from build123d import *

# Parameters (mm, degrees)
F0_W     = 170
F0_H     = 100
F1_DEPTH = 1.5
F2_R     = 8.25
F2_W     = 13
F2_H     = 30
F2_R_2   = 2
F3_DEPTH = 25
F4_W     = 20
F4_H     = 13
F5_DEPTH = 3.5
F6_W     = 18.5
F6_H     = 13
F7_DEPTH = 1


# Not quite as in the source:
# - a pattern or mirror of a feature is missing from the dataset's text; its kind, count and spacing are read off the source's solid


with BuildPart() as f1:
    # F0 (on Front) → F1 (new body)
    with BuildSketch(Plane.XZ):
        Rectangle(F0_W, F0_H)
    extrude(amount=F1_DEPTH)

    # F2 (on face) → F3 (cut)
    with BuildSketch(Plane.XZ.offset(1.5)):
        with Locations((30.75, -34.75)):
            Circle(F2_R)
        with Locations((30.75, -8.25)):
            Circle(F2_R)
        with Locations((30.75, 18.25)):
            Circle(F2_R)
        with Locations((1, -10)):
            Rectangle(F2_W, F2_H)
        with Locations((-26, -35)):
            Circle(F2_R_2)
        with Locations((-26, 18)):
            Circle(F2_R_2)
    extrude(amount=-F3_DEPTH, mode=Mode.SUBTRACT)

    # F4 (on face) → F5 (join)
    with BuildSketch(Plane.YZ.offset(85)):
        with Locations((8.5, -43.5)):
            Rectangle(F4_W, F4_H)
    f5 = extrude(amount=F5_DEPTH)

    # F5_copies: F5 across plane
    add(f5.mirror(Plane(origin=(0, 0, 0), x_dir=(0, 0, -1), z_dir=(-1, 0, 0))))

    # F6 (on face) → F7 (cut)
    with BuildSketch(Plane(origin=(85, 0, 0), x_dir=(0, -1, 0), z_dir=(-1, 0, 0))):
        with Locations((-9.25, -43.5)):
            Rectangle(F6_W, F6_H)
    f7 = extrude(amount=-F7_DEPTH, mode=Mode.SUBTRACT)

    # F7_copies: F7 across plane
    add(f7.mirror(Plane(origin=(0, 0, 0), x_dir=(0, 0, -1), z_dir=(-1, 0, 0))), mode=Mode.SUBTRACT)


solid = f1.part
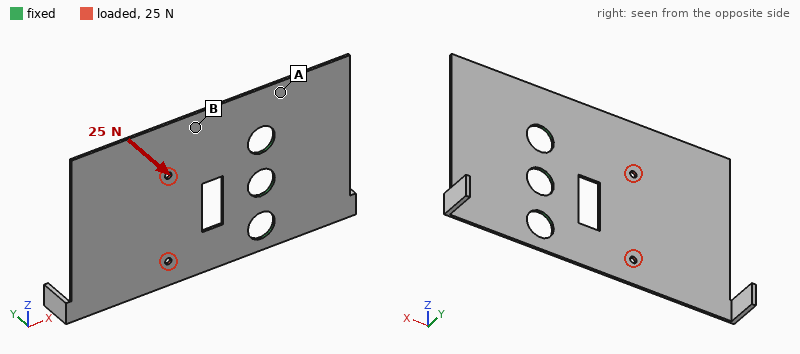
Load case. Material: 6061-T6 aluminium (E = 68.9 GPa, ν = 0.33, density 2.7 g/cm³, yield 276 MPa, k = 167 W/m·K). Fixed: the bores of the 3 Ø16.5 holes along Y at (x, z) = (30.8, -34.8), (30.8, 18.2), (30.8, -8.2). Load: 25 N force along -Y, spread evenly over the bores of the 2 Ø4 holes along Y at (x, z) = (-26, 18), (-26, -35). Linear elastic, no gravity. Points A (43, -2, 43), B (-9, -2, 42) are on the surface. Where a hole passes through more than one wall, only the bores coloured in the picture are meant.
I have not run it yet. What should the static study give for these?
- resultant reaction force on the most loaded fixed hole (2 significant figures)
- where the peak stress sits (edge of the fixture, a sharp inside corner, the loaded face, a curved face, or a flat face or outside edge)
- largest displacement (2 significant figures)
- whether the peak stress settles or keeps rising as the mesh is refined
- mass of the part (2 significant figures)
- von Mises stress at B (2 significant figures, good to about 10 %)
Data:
11 N
a sharp inside corner
2.1 mm
keeps rising
68 g
15 MPa
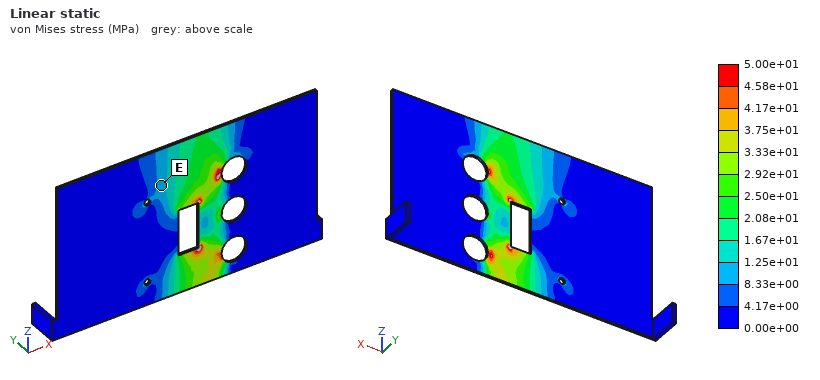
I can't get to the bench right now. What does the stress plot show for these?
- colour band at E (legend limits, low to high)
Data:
8.33e+00 to 1.25e+01 MPa
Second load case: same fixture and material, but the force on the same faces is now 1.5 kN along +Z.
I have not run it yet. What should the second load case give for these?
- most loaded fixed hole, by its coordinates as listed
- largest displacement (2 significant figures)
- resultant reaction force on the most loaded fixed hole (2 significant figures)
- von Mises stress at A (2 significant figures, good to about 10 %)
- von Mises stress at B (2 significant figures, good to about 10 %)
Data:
(30.8, 18.2)
84 µm
1.3 kN
14 MPa
13 MPa
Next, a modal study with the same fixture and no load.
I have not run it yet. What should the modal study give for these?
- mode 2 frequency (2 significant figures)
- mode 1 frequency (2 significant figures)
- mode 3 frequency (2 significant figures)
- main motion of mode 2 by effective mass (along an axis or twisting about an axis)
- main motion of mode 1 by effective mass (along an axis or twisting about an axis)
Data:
230 Hz
86 Hz
430 Hz
twisting about X
along Y
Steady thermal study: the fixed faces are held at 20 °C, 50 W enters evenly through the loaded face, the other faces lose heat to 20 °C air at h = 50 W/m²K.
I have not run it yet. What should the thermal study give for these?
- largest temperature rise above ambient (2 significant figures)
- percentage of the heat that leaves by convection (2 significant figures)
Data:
79 K
68 %
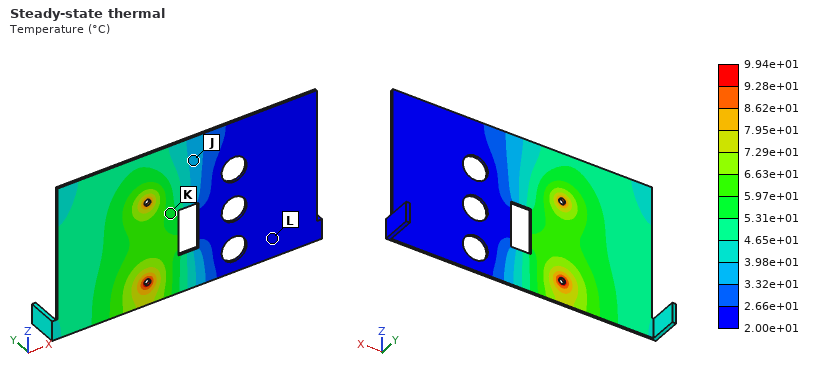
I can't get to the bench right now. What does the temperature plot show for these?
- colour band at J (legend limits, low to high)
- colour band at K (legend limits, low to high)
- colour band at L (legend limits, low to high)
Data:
3.32e+01 to 3.98e+01 °C
5.31e+01 to 5.97e+01 °C
2.00e+01 to 2.66e+01 °C
